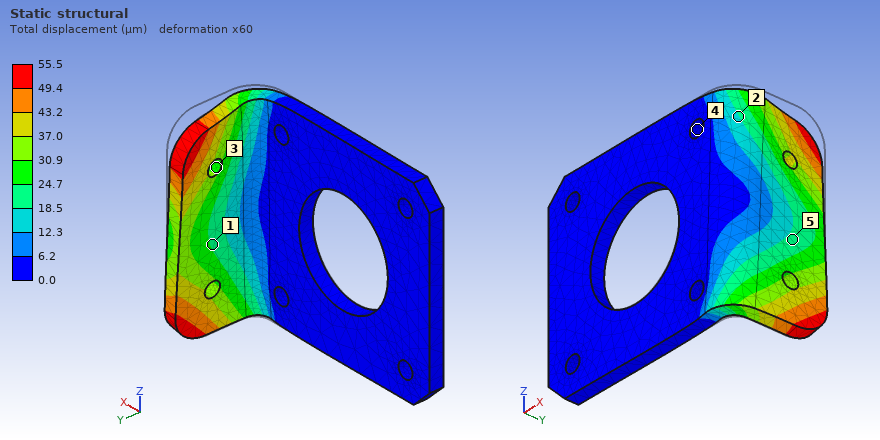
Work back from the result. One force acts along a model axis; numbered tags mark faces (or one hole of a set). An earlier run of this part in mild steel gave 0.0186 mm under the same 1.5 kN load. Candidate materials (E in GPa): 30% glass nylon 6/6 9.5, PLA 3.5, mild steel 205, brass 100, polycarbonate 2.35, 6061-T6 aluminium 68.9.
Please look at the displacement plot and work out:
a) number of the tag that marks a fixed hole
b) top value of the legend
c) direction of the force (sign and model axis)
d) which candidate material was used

4
55.5 µm
-Z
6061-T6 aluminium
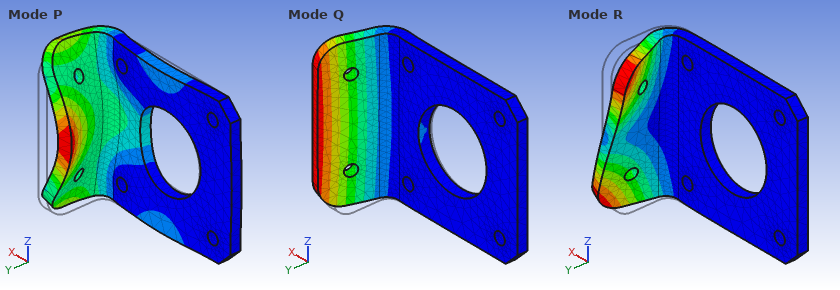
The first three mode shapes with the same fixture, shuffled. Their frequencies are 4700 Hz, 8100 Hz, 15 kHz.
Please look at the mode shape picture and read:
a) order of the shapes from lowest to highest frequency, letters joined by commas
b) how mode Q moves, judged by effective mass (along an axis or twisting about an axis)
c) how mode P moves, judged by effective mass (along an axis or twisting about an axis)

Q, R, P
along X
along Y
